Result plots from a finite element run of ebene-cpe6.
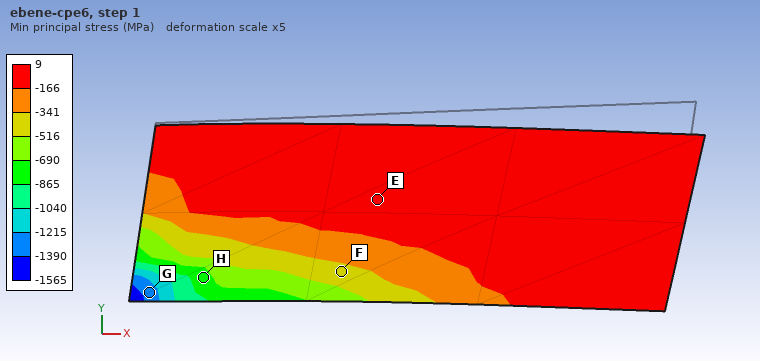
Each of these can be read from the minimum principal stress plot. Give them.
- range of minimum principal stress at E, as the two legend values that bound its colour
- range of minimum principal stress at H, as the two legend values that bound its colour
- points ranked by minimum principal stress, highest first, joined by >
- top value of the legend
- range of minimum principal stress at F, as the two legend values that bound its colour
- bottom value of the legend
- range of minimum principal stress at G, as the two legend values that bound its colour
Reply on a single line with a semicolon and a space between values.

-166 to 9 MPa; -865 to -690 MPa; E > F > H > G; 9 MPa; -516 to -341 MPa; -1565 MPa; -1390 to -1215 MPa
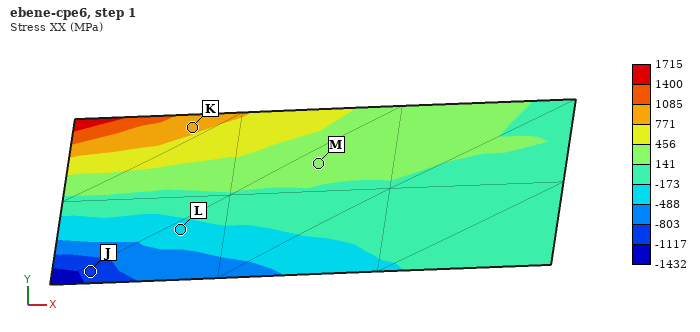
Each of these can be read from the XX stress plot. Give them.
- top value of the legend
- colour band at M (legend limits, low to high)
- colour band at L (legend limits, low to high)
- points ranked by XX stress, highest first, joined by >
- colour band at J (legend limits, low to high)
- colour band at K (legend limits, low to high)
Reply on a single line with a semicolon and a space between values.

1715 MPa; 141 to 456 MPa; -488 to -173 MPa; K > M > L > J; -1117 to -803 MPa; 771 to 1085 MPa
